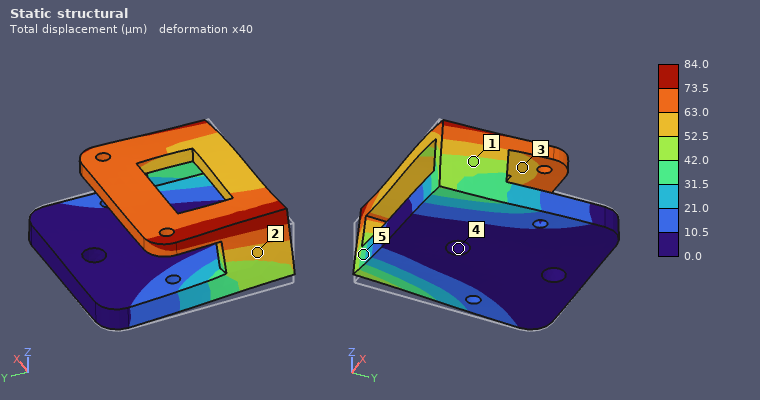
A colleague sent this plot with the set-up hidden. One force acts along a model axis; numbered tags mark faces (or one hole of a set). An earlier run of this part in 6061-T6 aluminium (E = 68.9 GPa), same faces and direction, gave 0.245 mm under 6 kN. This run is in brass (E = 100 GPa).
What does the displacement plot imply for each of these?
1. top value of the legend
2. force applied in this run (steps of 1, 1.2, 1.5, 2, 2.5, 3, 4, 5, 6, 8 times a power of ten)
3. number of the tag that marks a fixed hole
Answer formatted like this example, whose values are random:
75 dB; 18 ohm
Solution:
84.0 µm; 3 kN; 4
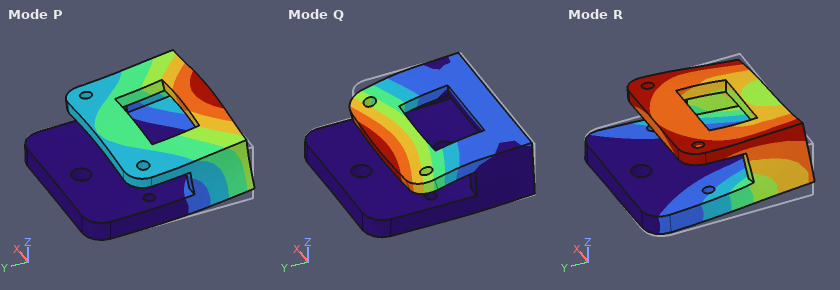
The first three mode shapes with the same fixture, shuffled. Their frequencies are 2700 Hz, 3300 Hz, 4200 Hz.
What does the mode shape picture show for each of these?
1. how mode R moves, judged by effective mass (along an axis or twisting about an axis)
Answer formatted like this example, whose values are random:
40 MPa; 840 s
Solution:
along X
